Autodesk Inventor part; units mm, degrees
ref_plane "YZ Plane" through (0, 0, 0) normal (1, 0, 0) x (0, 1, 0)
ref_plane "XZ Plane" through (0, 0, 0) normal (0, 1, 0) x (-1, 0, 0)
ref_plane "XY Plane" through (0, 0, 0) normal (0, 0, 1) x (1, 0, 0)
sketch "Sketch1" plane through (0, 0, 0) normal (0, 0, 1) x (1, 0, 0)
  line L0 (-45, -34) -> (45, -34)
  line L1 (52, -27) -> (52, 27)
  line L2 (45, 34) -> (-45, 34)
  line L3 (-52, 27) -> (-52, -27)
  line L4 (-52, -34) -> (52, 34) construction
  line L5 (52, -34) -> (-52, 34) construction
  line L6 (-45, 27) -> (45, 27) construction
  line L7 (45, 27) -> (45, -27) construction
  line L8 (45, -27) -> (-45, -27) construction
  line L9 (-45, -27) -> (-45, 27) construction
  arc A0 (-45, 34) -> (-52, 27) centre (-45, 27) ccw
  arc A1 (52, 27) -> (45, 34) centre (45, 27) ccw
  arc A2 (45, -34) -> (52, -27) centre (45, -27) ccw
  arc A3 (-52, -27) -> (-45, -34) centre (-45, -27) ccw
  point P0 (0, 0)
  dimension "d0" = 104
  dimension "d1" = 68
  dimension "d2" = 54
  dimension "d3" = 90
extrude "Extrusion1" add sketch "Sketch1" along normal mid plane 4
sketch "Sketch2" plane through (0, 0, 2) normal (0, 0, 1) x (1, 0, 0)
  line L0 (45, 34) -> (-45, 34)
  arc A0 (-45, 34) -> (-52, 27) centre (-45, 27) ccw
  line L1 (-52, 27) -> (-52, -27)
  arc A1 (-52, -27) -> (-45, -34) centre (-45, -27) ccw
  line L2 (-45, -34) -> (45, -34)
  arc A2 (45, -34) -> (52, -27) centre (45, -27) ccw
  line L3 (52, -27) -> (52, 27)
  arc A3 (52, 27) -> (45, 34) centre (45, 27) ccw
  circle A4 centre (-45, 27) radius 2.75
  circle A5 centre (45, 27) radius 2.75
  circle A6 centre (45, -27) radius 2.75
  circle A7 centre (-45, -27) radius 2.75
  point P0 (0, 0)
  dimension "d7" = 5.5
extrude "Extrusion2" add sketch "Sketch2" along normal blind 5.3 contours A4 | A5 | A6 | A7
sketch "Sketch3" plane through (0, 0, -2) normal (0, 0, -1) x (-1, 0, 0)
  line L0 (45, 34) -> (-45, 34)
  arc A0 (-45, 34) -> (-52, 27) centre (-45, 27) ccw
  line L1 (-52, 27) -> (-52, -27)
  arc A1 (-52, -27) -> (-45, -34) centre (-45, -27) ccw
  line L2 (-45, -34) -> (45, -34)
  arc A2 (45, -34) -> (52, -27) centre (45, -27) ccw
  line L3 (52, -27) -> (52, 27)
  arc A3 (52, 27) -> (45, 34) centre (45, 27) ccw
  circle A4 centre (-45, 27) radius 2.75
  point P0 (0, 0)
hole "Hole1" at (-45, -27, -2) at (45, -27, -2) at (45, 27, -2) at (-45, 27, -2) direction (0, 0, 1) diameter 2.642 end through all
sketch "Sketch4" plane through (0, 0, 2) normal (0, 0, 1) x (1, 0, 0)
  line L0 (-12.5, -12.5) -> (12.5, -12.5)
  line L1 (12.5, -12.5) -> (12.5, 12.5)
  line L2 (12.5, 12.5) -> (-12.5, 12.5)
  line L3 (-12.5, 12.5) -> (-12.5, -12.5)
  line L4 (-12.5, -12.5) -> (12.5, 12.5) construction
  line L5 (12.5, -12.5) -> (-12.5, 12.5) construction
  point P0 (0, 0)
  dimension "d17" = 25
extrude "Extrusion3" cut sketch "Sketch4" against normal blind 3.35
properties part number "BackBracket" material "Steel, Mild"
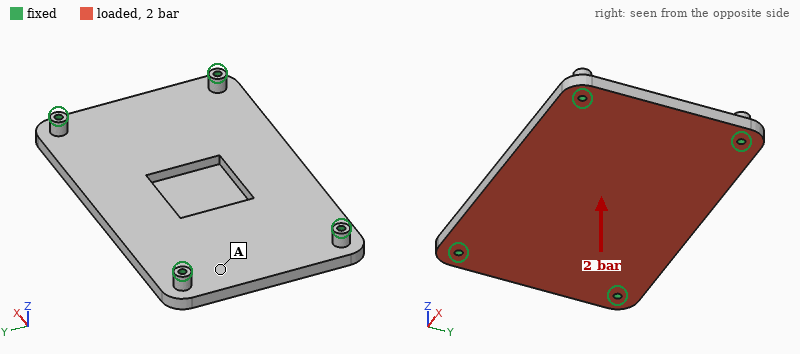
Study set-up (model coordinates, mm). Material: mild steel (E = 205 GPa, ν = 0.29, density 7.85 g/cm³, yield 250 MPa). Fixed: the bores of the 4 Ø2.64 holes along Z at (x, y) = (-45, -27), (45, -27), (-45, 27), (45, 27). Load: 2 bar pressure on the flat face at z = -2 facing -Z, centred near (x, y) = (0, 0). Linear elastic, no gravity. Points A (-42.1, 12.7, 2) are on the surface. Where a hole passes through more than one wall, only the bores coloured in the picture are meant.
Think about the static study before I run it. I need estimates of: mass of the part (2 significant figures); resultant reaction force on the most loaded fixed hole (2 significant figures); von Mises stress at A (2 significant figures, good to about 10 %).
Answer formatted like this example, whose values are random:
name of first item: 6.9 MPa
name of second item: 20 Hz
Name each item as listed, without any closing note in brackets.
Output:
mass of the part: 210 g
resultant reaction force on the most loaded fixed hole: 390 N
von Mises stress at A: 21 MPa
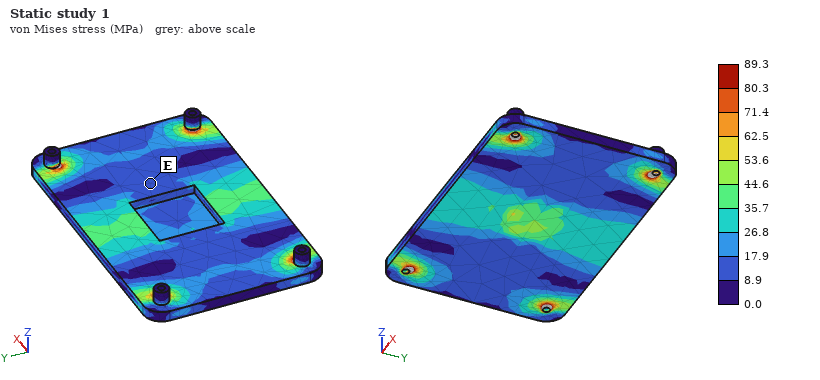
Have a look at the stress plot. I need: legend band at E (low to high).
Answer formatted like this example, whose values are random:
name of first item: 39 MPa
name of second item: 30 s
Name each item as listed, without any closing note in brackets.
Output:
legend band at E: 8.9 to 17.9 MPa
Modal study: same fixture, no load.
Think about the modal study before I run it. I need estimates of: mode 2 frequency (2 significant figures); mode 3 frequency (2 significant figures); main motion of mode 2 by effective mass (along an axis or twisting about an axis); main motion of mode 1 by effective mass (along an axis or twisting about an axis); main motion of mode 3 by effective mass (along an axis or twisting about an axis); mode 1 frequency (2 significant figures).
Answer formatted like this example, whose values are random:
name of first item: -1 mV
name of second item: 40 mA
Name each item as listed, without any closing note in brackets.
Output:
mode 2 frequency: 3300 Hz
mode 3 frequency: 5200 Hz
main motion of mode 2 by effective mass: twisting about X
main motion of mode 1 by effective mass: along Z
main motion of mode 3 by effective mass: twisting about Y
mode 1 frequency: 2200 Hz
